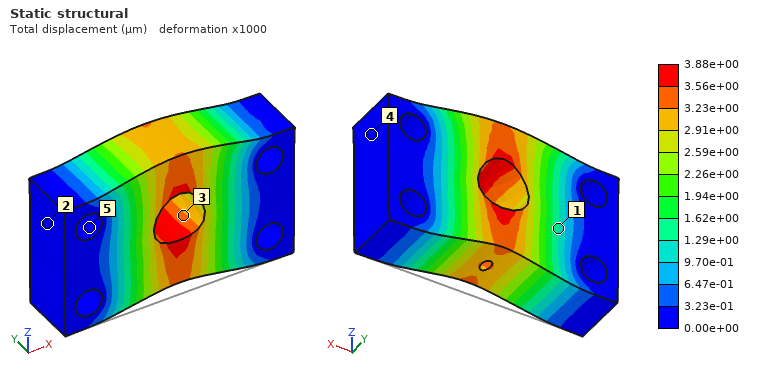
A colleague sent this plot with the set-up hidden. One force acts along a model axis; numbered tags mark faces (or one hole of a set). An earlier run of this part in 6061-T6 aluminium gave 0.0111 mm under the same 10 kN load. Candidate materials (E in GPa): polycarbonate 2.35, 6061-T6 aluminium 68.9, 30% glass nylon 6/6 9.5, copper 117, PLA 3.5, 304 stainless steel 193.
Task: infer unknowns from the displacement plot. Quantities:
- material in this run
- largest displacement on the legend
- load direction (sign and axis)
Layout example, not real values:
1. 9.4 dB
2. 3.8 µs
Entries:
1. 304 stainless steel
2. 3.88e+00 µm
3. +Z
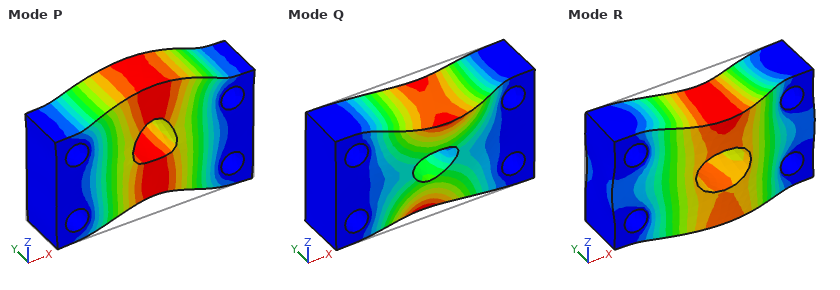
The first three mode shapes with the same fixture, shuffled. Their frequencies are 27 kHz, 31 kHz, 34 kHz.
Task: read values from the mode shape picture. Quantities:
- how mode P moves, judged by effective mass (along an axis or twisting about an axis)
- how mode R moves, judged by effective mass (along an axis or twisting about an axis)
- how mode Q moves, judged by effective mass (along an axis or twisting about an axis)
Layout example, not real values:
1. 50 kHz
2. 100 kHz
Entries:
1. along Z
2. along Y
3. twisting about X
